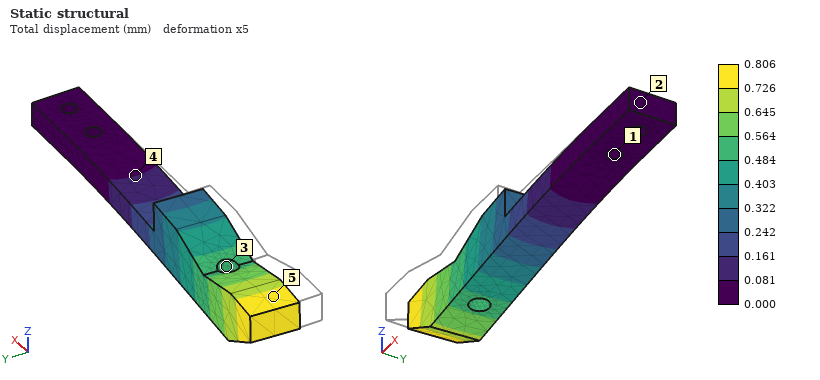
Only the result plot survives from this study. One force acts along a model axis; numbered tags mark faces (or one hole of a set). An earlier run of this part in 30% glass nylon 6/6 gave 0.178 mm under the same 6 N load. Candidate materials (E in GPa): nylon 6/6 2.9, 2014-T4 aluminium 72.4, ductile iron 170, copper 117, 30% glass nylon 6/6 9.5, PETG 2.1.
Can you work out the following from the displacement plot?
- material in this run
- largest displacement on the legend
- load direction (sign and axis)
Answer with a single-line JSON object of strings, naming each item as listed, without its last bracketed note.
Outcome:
{"material in this run": "PETG", "largest displacement on the legend": "0.806 mm", "load direction": "+Y"}
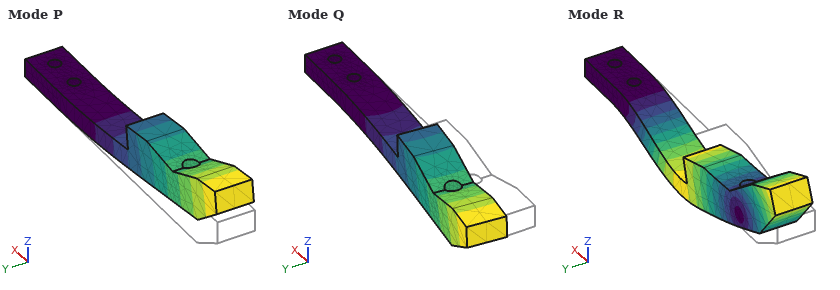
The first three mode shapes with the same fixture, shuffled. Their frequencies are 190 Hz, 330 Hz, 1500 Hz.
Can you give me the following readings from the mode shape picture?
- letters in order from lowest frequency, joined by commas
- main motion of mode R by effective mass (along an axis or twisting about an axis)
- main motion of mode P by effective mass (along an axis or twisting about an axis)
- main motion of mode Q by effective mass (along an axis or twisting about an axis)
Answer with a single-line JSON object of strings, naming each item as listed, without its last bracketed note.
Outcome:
{"letters in order from lowest frequency, joined by commas": "P, Q, R", "main motion of mode R by effective mass": "along Z", "main motion of mode P by effective mass": "along Z", "main motion of mode Q by effective mass": "along Y"}
